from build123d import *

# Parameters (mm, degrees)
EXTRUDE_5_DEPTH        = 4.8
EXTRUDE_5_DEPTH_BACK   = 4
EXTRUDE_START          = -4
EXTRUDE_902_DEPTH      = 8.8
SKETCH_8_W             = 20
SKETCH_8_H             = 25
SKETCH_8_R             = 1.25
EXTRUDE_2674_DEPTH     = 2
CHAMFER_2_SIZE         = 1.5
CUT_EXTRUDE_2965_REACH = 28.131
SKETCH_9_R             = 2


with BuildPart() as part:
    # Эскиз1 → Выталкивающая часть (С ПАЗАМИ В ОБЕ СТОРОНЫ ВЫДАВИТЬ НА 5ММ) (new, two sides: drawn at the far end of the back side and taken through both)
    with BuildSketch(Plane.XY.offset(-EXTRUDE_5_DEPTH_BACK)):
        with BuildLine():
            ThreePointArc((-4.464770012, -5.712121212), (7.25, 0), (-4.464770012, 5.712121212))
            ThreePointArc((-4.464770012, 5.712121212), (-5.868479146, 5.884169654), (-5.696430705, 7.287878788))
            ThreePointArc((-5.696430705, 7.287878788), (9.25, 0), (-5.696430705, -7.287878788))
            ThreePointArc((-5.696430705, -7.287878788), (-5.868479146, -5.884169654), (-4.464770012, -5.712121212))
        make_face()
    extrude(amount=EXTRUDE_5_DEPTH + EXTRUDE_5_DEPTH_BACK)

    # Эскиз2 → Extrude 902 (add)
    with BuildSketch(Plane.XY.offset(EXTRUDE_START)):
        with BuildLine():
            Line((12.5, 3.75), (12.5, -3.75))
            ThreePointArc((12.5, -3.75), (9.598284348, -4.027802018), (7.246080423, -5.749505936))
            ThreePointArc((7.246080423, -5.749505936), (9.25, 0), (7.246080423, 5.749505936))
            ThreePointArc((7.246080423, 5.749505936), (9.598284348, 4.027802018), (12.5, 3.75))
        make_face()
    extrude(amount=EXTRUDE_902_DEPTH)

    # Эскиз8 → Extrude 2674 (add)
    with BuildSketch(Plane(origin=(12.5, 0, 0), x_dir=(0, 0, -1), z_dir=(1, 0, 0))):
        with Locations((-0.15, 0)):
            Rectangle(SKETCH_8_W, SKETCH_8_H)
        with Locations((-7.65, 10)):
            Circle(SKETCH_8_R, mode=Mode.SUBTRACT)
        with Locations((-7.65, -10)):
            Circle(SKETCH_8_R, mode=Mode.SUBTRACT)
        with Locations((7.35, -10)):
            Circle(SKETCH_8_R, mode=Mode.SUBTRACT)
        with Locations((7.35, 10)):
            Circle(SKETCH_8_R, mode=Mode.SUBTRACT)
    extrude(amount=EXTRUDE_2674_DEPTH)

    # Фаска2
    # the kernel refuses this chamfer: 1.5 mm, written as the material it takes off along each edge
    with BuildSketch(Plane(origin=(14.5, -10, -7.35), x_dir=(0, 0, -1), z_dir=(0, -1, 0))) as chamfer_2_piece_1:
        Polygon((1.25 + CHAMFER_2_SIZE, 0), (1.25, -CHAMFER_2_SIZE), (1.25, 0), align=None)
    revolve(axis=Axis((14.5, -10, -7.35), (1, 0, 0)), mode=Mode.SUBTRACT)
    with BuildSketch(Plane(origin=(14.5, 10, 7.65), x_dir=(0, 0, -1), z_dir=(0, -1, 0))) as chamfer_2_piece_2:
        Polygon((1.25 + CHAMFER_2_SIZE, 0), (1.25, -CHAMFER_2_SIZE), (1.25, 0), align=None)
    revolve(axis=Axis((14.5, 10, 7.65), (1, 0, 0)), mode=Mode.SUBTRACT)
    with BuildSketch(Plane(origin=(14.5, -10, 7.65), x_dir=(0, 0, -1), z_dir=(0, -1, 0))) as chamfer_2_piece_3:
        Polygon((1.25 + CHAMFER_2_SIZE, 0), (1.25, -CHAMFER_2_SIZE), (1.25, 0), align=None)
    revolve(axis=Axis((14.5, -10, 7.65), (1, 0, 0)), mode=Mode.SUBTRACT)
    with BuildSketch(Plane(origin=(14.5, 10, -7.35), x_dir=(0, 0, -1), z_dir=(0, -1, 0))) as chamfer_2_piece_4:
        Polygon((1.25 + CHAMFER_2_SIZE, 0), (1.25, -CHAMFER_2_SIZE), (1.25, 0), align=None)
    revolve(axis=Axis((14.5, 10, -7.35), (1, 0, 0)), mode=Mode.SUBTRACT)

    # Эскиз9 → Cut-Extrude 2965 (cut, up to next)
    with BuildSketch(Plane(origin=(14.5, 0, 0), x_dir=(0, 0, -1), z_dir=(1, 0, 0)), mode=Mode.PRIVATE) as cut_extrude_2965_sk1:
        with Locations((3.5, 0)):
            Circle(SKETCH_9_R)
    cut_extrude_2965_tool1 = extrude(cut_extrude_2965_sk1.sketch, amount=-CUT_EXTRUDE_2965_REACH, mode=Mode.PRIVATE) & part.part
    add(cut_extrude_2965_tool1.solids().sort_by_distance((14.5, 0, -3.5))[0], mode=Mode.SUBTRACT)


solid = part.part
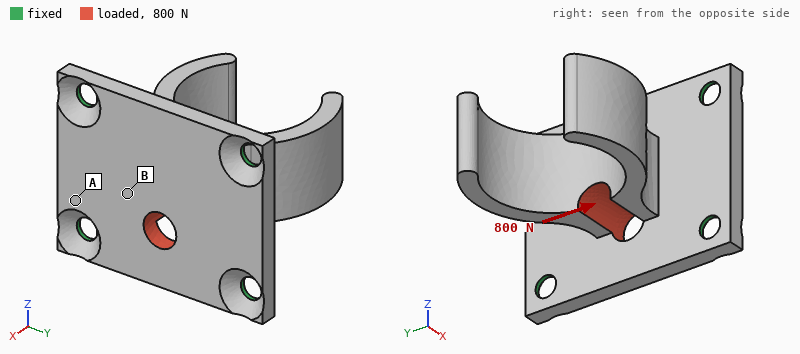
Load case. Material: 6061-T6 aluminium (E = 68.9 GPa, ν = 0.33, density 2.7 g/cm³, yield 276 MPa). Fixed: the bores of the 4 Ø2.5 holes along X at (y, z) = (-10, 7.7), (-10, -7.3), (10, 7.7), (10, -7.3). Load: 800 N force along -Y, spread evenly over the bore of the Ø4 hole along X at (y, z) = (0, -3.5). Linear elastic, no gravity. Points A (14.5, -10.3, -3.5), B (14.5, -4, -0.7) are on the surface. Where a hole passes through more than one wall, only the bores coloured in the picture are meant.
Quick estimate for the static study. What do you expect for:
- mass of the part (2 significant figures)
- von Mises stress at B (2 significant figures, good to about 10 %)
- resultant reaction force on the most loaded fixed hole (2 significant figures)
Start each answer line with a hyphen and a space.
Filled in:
- 4.8 g
- 36 MPa
- 240 N
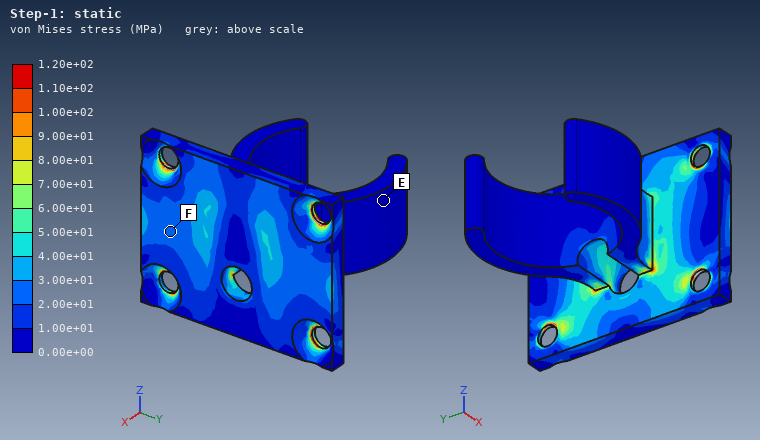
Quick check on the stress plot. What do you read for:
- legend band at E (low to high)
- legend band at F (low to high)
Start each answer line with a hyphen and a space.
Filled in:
- 0.00e+00 to 1.00e+01 MPa
- 2.00e+01 to 3.00e+01 MPa
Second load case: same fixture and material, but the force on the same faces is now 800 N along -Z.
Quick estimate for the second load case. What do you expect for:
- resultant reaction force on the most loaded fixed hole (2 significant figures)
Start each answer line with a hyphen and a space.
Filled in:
- 210 N
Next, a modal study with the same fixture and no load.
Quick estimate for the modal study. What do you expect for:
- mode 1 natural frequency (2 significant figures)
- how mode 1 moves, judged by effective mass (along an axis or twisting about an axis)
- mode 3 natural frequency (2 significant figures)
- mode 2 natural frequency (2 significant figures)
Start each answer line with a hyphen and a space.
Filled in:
- 5300 Hz
- along Y
- 6900 Hz
- 6700 Hz
